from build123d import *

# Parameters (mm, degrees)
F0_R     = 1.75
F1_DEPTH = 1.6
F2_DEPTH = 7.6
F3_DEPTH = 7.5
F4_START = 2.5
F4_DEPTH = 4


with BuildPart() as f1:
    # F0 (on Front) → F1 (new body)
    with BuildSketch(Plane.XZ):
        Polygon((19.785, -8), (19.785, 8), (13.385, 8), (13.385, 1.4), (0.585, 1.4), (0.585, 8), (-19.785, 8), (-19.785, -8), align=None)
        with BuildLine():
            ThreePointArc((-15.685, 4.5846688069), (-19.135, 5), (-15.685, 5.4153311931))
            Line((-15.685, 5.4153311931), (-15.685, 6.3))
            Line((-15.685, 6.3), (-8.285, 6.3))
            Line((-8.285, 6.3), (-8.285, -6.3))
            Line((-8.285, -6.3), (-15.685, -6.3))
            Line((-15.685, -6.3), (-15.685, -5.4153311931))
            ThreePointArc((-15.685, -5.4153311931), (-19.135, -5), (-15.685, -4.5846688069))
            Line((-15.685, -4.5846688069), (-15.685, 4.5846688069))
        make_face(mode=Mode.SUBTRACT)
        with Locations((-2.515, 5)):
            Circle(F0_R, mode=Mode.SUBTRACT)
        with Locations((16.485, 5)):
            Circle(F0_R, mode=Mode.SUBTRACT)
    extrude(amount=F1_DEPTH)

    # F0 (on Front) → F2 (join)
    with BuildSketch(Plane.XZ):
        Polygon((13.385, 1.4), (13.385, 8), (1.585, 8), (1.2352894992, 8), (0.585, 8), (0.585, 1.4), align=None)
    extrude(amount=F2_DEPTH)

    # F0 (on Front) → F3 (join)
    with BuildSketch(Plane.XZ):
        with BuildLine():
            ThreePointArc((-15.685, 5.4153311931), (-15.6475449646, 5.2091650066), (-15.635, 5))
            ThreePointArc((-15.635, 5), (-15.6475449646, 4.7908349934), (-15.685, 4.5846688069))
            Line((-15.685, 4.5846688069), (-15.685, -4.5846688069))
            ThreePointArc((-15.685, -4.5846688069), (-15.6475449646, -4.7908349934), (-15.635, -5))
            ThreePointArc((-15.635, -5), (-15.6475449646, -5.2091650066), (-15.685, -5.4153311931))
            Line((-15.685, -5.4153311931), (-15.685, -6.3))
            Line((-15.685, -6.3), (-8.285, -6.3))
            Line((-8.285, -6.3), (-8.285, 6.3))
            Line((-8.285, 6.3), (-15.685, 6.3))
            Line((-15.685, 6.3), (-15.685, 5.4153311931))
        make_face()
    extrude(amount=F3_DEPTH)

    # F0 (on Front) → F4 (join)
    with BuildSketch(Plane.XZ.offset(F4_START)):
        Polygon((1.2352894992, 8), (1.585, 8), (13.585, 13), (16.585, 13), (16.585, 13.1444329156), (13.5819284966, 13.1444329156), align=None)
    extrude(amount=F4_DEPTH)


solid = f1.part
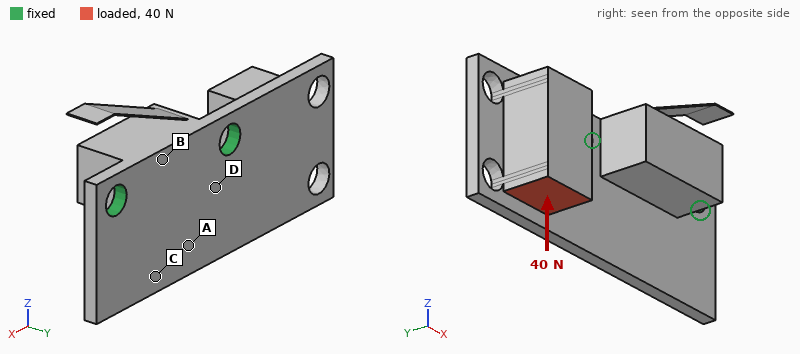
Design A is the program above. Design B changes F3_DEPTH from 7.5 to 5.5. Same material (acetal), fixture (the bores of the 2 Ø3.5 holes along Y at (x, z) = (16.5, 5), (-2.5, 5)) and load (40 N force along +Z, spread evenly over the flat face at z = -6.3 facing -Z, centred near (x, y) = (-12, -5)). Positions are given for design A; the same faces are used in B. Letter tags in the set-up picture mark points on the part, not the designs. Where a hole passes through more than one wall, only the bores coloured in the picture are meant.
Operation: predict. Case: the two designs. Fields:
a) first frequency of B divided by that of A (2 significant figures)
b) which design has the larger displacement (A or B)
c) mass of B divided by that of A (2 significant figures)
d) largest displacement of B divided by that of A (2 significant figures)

1.0
A
0.91
0.74
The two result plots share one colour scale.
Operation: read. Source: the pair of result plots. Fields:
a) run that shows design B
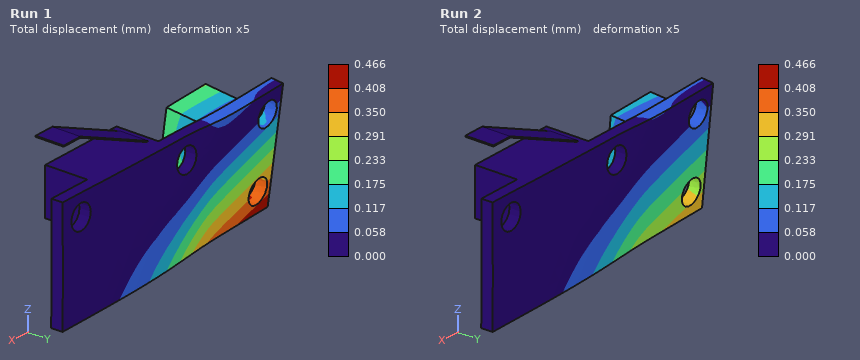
Run 2
